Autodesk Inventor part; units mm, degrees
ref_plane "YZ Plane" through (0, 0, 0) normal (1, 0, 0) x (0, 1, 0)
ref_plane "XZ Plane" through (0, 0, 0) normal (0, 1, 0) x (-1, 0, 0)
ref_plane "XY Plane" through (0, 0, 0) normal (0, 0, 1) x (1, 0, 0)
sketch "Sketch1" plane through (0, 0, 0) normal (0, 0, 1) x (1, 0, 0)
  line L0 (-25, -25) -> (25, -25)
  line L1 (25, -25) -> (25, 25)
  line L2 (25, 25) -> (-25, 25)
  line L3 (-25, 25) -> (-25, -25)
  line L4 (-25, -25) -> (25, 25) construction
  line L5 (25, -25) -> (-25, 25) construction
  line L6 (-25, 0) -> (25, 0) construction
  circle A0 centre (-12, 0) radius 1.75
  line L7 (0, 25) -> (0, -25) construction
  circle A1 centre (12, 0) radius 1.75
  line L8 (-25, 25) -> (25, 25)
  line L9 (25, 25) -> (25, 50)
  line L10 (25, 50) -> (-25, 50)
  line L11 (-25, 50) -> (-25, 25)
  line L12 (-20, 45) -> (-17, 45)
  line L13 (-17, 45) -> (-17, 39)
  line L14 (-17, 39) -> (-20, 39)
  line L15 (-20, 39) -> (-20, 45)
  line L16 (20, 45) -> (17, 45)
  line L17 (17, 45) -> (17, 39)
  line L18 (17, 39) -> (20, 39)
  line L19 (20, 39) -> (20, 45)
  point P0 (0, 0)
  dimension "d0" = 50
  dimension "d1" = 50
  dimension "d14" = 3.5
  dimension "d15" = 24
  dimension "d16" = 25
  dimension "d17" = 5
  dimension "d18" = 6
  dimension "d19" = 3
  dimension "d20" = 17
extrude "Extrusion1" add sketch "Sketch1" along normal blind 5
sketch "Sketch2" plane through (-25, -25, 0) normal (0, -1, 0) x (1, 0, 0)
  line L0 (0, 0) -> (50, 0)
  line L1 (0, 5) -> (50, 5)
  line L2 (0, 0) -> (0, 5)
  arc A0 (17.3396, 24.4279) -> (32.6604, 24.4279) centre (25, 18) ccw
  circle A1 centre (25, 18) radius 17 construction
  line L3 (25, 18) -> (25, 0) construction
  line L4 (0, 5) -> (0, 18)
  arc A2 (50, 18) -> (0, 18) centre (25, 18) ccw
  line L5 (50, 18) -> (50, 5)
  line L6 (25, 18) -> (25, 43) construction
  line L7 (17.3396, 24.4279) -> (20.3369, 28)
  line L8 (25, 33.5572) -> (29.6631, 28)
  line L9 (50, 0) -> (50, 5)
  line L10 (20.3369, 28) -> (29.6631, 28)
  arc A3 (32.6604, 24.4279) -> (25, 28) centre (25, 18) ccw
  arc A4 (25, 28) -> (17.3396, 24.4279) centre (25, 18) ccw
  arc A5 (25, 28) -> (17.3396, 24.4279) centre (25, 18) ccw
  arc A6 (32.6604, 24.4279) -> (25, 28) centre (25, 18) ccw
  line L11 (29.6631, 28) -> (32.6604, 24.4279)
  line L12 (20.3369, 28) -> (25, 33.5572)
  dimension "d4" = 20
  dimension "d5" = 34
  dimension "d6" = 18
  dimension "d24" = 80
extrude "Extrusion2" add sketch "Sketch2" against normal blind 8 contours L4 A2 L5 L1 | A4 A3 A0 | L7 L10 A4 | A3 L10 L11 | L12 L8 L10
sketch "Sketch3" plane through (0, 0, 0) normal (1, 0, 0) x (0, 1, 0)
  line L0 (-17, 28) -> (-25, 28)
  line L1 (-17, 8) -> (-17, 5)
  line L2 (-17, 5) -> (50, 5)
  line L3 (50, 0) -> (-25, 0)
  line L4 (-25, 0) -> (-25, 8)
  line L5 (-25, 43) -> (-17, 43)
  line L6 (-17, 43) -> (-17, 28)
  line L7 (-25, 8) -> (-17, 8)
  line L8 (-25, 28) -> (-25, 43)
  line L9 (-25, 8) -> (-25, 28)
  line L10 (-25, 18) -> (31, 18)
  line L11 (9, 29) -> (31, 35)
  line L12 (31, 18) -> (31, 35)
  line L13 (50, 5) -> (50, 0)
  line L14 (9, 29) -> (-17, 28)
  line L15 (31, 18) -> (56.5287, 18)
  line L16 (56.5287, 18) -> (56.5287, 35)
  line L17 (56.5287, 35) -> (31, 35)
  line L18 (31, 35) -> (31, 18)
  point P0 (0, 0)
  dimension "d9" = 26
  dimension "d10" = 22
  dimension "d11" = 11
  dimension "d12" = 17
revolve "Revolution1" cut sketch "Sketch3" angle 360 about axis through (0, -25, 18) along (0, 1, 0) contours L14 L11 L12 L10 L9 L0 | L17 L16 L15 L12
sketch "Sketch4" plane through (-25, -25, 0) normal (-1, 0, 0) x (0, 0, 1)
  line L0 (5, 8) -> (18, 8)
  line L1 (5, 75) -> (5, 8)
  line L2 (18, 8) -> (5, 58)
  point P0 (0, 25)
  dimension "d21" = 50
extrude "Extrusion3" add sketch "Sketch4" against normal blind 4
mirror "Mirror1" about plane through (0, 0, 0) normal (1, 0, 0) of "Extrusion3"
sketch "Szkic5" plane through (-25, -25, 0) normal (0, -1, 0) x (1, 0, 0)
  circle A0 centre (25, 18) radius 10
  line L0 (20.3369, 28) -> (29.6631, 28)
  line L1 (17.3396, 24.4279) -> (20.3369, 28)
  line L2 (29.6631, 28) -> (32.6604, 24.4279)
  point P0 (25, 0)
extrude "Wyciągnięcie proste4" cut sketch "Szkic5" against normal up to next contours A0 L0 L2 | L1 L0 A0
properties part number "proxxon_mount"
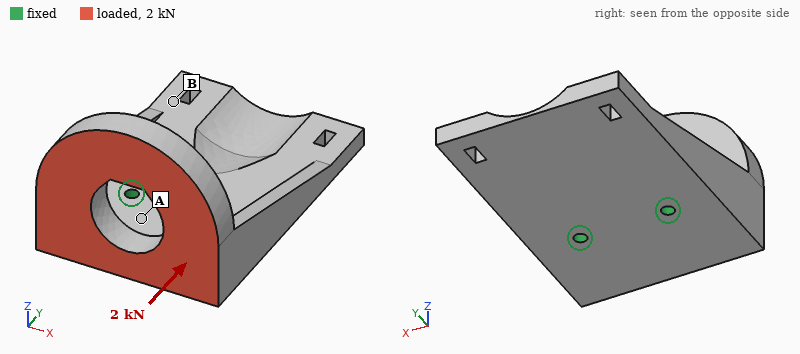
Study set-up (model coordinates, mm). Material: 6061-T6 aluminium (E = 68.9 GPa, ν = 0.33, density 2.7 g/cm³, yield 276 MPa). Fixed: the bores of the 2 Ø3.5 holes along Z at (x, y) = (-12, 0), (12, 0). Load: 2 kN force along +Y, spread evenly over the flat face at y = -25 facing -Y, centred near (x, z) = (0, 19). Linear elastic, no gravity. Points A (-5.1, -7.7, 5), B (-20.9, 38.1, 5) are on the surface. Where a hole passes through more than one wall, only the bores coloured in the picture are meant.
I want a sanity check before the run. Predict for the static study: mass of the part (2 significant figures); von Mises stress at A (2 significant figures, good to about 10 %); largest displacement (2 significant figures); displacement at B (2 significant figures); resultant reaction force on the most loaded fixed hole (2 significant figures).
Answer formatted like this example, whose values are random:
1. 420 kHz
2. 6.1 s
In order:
1. 81 g
2. 56 MPa
3. 0.39 mm
4. 0.18 mm
5. 1.0 kN
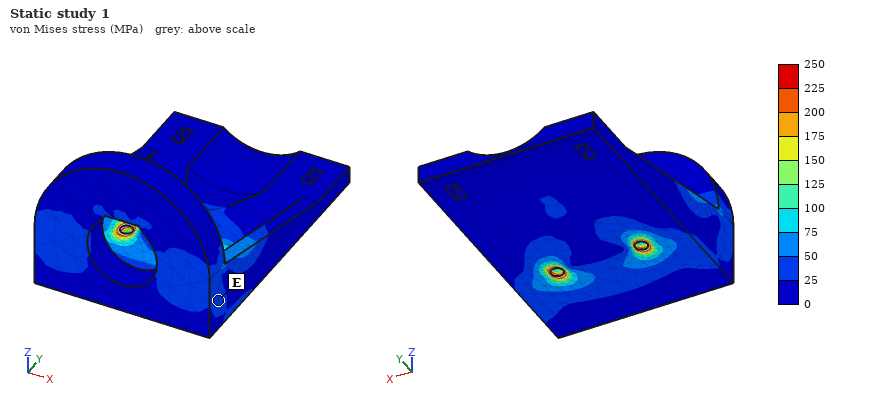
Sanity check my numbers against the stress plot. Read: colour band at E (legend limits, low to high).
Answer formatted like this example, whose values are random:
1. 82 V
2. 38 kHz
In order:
1. 25 to 50 MPa
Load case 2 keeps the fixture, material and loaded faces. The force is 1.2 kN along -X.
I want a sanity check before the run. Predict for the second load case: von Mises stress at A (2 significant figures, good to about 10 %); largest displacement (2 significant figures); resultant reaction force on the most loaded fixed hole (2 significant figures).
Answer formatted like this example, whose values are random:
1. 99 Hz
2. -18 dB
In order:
1. 33 MPa
2. 81 µm
3. 1.4 kN
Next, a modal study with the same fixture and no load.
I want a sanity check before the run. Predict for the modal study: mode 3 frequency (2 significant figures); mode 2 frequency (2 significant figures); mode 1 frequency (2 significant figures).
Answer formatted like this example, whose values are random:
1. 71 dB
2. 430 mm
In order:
1. 3200 Hz
2. 3100 Hz
3. 1700 Hz
